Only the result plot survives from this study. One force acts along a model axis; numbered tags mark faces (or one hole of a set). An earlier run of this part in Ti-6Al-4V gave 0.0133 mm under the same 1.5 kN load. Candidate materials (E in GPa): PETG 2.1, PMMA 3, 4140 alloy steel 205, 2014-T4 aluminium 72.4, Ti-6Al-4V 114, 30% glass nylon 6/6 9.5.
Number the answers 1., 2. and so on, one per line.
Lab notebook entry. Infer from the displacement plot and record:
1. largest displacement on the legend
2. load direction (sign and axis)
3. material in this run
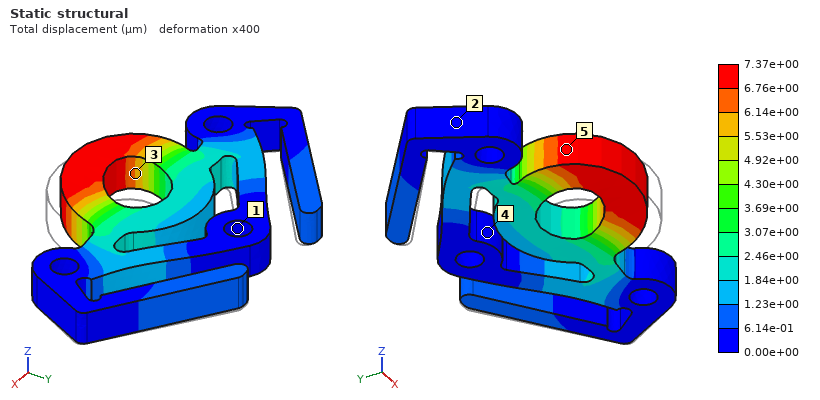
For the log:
1. 7.37e+00 µm
2. -X
3. 4140 alloy steel
